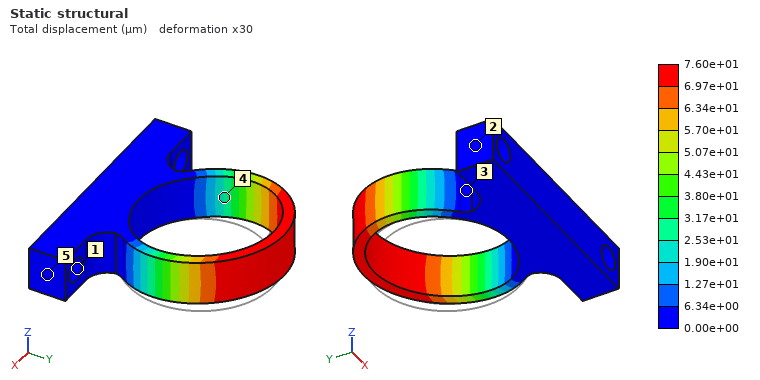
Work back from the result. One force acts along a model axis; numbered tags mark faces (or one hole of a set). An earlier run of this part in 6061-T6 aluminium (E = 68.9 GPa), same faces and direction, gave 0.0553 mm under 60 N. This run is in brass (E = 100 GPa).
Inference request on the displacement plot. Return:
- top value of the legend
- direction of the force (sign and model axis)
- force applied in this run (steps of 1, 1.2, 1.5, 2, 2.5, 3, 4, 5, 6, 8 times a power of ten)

7.60e+01 µm
-X
120 N
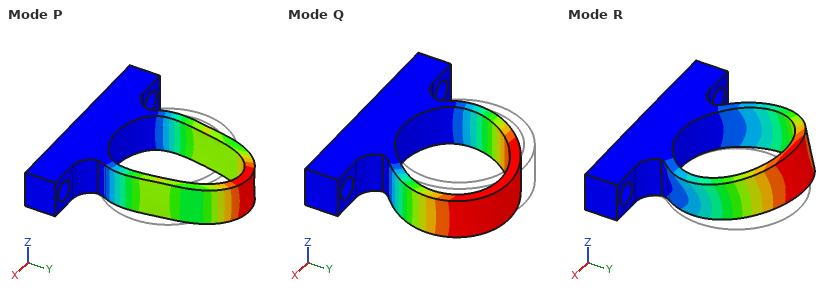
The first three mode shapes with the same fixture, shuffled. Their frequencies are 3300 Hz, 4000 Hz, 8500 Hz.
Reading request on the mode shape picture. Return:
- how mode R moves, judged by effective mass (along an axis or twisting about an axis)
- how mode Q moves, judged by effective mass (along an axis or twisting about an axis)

along Z
along X
